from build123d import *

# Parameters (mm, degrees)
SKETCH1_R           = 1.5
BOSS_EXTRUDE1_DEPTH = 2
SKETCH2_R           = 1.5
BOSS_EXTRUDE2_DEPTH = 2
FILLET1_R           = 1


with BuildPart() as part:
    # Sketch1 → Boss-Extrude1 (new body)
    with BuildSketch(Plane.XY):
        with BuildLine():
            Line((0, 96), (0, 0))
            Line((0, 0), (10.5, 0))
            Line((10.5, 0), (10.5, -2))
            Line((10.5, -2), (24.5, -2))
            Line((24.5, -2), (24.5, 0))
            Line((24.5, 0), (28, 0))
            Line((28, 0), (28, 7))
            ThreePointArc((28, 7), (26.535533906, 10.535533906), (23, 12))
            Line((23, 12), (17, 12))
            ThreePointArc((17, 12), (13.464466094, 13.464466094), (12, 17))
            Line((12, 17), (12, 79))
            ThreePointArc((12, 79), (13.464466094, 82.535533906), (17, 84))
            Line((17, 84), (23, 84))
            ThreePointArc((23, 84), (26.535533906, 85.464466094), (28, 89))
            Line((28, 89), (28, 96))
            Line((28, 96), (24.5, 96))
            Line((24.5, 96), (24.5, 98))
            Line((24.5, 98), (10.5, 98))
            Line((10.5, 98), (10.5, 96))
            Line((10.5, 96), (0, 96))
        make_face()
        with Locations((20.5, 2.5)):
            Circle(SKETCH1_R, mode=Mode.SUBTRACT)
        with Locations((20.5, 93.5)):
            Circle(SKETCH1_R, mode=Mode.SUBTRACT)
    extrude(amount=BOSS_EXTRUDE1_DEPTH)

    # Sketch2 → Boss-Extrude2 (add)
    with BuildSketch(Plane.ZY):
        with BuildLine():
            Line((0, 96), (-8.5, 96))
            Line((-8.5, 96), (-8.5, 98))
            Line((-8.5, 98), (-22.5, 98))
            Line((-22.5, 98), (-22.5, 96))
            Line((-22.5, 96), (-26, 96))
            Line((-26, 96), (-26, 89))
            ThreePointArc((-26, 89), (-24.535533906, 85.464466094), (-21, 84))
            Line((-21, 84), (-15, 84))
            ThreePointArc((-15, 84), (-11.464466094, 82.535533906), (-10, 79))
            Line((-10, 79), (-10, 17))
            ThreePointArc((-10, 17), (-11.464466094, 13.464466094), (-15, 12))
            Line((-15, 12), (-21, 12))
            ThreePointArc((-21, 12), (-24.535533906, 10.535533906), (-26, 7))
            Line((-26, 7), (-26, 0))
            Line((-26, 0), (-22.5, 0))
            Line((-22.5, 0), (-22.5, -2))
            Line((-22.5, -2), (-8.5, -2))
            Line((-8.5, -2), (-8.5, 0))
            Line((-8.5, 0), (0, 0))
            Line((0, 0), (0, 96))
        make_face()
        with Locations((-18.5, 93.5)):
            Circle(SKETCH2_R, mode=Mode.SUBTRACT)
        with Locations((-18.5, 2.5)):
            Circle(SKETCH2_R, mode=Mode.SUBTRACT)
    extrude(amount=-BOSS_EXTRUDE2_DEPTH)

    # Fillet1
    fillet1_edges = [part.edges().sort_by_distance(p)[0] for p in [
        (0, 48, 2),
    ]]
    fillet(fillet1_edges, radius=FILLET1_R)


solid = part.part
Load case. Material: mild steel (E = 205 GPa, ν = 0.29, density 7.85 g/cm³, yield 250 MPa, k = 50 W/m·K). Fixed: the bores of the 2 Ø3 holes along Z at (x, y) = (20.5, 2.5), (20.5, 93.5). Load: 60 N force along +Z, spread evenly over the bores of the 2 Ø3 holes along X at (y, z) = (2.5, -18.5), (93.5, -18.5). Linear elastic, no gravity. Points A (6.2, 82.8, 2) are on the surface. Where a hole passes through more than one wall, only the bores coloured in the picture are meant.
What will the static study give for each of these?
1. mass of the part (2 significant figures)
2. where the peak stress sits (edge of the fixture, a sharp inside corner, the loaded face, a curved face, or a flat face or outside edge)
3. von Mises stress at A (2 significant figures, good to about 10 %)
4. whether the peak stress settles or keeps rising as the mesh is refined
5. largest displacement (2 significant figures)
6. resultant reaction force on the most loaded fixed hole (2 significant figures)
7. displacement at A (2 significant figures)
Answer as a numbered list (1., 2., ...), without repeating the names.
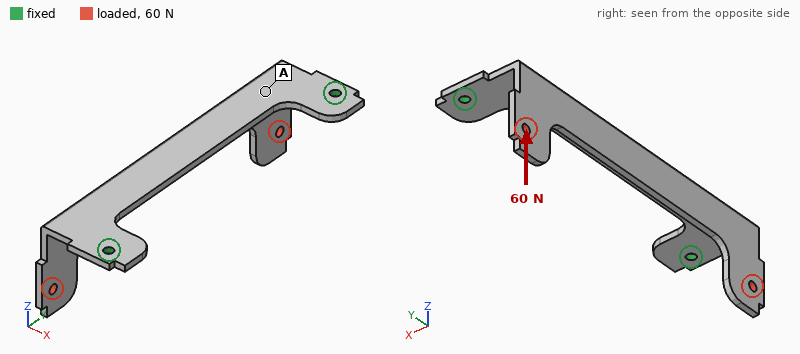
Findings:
1. 46 g
2. edge of the fixture
3. 8.7 MPa
4. keeps rising
5. 84 µm
6. 30 N
7. 24 µm
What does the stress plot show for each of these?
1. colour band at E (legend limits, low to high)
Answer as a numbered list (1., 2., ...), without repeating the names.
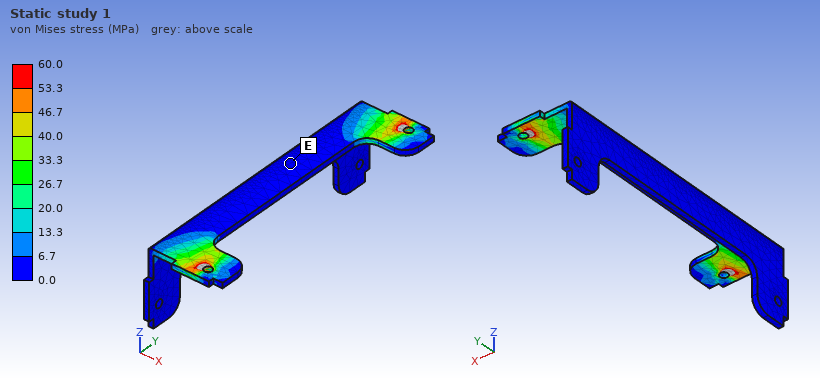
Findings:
1. 0.0 to 6.7 MPa
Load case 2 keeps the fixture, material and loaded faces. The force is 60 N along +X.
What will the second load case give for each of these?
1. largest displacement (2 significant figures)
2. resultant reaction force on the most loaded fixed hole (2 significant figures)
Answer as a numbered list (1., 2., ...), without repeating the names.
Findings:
1. 0.19 mm
2. 30 N
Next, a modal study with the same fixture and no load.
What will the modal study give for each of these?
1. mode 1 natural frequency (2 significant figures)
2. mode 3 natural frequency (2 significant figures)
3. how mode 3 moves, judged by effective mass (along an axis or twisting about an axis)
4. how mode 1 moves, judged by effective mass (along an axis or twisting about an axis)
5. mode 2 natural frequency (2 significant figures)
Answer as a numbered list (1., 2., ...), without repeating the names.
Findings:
1. 890 Hz
2. 2300 Hz
3. along Z
4. along Z
5. 1400 Hz
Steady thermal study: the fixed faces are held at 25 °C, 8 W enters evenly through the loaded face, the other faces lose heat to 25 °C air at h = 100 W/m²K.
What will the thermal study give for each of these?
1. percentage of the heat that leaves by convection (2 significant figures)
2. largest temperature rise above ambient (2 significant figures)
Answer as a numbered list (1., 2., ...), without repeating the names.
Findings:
1. 85 %
2. 46 K
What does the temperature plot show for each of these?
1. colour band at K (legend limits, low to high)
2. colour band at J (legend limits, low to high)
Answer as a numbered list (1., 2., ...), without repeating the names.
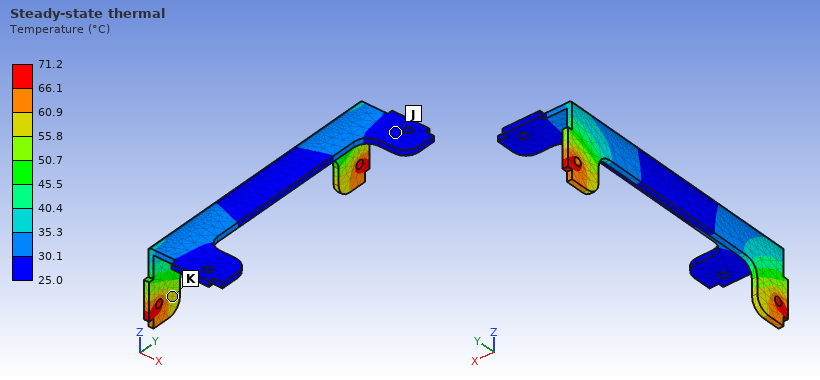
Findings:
1. 55.8 to 60.9 °C
2. 25.0 to 30.1 °C
